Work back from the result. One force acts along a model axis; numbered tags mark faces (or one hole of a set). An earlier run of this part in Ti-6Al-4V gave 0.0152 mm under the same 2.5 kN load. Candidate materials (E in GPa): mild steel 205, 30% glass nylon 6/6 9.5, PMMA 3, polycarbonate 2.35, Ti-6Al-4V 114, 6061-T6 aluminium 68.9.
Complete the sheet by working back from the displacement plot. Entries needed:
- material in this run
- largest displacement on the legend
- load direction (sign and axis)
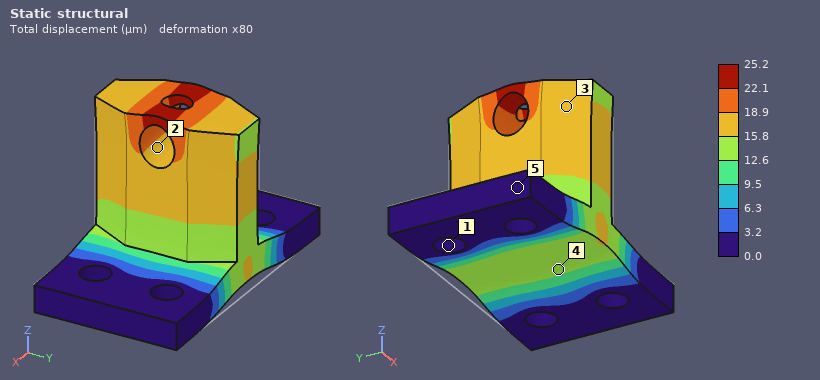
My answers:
6061-T6 aluminium
25.2 µm
+Z
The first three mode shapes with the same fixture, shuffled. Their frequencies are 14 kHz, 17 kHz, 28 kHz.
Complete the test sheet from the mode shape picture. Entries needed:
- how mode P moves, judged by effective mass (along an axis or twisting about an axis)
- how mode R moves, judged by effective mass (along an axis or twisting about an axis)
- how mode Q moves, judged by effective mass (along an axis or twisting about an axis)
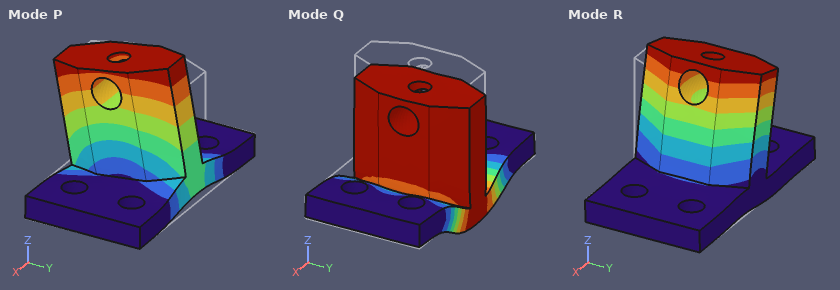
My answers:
along Y
along X
along Z
